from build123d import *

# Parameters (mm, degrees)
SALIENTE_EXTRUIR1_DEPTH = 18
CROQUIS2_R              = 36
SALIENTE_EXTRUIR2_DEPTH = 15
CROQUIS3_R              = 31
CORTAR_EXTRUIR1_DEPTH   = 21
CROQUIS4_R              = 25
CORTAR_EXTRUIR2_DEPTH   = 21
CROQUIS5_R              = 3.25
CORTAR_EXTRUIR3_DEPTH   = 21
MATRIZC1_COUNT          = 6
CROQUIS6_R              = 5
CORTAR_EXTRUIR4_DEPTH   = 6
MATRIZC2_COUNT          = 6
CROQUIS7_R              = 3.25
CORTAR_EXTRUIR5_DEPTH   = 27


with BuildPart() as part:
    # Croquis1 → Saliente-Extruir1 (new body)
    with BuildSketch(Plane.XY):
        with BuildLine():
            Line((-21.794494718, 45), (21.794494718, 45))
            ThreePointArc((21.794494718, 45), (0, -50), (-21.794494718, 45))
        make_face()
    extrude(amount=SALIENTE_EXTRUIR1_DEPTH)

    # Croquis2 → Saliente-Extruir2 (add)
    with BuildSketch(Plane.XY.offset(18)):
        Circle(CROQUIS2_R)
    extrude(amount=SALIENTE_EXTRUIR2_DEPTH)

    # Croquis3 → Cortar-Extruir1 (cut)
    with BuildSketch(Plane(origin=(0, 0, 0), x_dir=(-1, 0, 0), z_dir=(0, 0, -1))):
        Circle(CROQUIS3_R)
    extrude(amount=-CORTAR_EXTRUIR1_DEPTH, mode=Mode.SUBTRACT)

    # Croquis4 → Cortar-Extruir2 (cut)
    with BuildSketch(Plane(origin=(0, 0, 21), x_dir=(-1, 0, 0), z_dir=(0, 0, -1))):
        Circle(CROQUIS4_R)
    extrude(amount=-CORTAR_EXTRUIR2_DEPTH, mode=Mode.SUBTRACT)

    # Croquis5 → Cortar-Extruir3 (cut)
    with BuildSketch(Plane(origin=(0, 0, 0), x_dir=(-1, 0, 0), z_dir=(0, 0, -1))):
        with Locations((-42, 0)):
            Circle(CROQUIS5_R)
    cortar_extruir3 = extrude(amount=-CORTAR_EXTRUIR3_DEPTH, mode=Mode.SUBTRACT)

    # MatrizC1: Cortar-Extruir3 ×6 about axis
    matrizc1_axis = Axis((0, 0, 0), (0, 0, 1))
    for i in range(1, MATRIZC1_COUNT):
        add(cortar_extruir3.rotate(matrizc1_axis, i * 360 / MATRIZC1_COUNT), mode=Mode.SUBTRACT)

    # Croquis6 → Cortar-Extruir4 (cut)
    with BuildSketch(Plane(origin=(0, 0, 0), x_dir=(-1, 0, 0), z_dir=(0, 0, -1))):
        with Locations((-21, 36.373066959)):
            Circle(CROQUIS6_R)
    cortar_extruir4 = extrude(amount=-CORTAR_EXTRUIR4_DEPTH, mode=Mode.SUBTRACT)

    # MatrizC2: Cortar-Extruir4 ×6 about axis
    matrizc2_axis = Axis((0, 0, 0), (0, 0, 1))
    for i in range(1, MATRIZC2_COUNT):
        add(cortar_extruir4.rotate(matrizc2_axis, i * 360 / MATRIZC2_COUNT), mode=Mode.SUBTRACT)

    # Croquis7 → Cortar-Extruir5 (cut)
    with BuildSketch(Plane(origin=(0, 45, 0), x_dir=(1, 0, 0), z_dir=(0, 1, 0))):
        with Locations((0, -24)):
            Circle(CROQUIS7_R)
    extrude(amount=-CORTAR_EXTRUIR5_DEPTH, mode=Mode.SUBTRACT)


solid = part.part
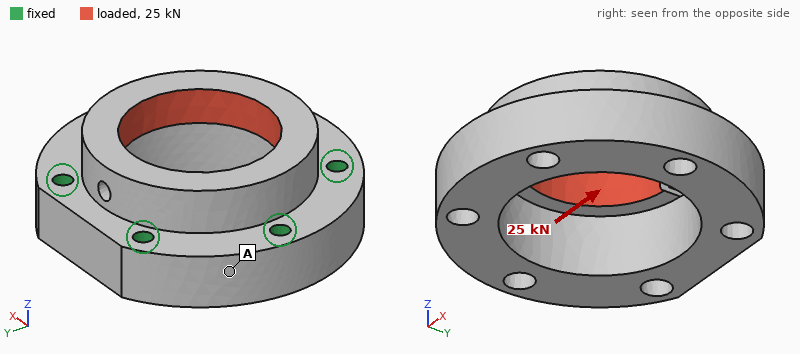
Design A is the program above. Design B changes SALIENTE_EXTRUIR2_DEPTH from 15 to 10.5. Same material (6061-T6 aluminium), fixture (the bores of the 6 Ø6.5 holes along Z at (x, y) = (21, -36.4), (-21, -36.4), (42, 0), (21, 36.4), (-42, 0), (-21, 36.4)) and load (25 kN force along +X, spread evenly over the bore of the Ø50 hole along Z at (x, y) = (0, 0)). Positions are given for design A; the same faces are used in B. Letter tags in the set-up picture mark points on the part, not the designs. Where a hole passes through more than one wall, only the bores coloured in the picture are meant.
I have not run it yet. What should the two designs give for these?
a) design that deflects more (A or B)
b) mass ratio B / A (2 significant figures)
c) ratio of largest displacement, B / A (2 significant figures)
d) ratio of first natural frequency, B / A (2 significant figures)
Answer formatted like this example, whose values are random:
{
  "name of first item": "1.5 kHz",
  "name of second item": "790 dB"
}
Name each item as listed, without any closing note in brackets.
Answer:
{
  "design that deflects more": "B",
  "mass ratio B / A": "0.91",
  "ratio of largest displacement, B / A": "1.2",
  "ratio of first natural frequency, B / A": "1.1"
}
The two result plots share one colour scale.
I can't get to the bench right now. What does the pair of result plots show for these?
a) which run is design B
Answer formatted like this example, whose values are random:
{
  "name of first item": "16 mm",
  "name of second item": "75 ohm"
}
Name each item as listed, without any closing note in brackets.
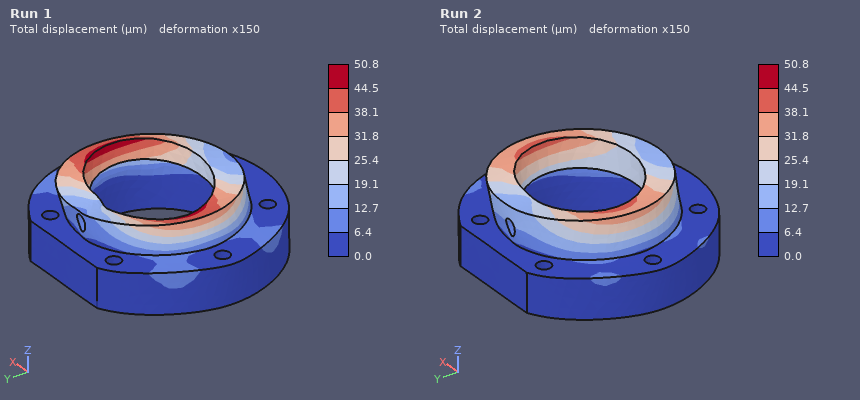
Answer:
{
  "which run is design B": "Run 1"
}
